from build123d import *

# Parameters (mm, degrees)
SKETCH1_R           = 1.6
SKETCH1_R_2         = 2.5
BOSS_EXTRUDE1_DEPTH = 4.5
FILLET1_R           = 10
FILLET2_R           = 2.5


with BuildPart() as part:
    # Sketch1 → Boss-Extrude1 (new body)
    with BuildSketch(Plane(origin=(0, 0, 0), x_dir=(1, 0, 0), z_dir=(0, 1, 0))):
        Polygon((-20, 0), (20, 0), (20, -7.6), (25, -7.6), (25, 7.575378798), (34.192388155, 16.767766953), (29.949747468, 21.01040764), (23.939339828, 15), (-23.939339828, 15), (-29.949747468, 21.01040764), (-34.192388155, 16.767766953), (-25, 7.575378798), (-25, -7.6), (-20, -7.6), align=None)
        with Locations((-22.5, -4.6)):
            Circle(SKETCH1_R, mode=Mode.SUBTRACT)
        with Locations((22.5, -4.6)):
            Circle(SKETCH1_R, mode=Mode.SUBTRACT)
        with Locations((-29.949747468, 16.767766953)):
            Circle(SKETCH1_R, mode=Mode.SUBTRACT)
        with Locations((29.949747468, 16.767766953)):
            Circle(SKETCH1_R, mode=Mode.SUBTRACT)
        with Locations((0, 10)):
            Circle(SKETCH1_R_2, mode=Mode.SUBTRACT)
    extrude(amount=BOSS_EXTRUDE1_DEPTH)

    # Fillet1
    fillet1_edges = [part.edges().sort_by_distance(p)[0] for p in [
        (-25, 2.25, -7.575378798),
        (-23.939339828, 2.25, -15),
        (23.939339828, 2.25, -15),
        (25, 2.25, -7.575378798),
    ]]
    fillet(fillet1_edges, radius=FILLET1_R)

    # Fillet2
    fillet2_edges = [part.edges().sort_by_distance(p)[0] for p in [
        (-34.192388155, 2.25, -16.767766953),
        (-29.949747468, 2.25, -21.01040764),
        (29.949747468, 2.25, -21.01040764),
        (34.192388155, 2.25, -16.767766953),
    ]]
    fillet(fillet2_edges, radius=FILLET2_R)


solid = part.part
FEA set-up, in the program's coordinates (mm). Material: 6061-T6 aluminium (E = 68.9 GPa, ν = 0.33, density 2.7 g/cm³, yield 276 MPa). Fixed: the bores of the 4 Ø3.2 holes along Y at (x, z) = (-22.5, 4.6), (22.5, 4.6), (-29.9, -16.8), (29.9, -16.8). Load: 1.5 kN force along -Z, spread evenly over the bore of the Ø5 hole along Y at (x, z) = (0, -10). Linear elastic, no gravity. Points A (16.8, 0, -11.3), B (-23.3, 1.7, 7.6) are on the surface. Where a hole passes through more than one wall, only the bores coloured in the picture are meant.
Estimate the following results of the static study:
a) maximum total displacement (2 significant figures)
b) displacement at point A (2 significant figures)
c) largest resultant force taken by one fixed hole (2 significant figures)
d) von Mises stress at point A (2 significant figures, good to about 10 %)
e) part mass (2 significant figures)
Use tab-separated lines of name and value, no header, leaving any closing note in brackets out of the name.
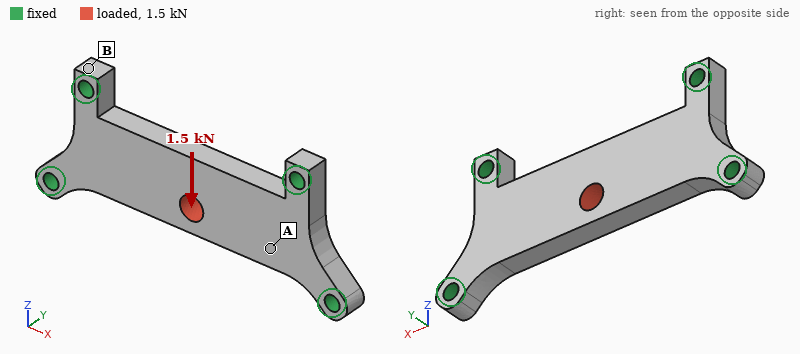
maximum total displacement	26 µm
displacement at point A	7.7 µm
largest resultant force taken by one fixed hole	690 N
von Mises stress at point A	21 MPa
part mass	11 g
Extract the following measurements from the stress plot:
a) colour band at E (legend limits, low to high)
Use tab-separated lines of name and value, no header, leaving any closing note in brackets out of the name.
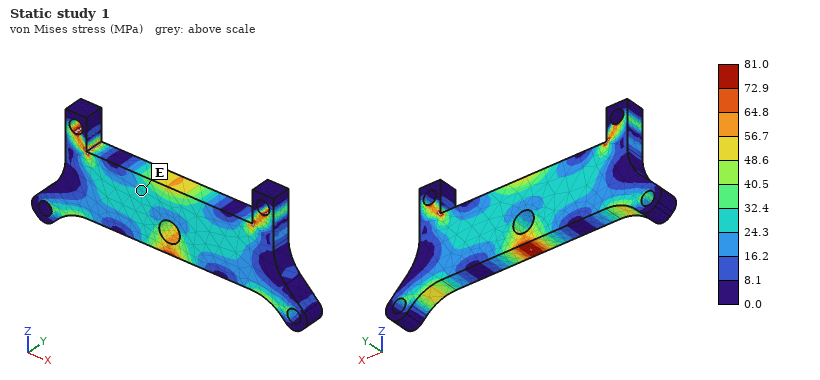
colour band at E	24.3 to 32.4 MPa
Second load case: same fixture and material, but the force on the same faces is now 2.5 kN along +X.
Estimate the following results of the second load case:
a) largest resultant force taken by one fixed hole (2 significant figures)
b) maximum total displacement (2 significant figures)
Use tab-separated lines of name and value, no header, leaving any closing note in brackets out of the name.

largest resultant force taken by one fixed hole	890 N
maximum total displacement	14 µm
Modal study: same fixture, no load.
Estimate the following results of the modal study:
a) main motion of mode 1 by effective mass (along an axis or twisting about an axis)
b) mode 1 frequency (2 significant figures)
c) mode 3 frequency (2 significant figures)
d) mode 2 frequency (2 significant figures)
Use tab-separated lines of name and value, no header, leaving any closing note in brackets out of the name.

main motion of mode 1 by effective mass	along Y
mode 1 frequency	6500 Hz
mode 3 frequency	18 kHz
mode 2 frequency	18 kHz
